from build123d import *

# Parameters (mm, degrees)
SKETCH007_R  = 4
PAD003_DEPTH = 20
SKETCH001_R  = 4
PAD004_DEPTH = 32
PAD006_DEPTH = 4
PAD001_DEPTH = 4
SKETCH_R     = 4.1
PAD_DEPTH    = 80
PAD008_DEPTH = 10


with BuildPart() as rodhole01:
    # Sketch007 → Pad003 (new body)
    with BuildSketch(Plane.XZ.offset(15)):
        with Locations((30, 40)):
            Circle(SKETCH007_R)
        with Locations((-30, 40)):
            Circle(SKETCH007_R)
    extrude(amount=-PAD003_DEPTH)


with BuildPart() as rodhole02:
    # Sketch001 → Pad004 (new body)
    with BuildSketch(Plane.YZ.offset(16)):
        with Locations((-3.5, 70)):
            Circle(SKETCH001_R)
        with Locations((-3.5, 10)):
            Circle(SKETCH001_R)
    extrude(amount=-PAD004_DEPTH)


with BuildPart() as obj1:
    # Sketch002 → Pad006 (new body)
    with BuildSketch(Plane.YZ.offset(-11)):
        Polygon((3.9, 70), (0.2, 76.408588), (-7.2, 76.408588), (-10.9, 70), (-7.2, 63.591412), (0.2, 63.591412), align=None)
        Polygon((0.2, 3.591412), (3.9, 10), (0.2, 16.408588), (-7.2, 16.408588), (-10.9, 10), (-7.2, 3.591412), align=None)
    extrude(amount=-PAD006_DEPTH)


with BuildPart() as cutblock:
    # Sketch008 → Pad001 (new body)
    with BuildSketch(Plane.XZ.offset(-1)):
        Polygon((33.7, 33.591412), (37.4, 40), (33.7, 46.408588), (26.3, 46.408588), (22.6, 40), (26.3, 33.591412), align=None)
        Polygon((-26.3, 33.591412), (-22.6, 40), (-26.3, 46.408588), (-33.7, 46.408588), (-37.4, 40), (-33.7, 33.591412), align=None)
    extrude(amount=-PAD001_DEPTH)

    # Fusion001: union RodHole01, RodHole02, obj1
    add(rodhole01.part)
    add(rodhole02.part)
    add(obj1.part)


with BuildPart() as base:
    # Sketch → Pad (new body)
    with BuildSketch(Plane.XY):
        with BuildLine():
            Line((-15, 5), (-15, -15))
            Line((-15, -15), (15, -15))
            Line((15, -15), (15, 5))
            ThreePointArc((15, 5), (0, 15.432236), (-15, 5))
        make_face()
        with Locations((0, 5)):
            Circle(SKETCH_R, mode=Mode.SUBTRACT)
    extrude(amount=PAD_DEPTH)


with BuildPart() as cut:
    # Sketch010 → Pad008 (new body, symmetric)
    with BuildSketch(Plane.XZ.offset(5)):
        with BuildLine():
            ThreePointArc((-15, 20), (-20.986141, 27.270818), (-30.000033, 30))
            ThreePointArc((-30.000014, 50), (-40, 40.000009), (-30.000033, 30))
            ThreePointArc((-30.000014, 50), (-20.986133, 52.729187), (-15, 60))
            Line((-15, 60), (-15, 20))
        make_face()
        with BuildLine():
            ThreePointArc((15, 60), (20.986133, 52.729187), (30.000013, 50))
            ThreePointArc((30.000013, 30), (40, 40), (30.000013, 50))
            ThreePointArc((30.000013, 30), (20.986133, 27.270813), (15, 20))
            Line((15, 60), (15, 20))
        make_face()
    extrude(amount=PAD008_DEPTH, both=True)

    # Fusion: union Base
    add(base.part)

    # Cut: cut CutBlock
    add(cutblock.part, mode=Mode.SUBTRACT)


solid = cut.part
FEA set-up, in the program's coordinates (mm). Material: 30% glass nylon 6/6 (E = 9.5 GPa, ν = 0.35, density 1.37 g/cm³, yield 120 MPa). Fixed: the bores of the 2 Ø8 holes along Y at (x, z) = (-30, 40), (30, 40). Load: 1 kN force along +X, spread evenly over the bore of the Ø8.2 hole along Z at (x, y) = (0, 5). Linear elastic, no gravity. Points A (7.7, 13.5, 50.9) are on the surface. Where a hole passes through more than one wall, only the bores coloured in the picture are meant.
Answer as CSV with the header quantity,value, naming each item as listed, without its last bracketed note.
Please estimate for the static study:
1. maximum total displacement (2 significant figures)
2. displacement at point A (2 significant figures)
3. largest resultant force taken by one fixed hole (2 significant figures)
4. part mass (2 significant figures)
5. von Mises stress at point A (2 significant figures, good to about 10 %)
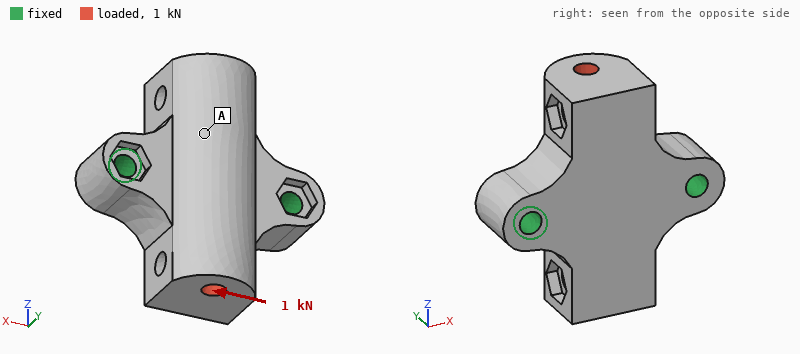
quantity,value
maximum total displacement,10 µm
displacement at point A,5.2 µm
largest resultant force taken by one fixed hole,540 N
part mass,110 g
von Mises stress at point A,0.64 MPa
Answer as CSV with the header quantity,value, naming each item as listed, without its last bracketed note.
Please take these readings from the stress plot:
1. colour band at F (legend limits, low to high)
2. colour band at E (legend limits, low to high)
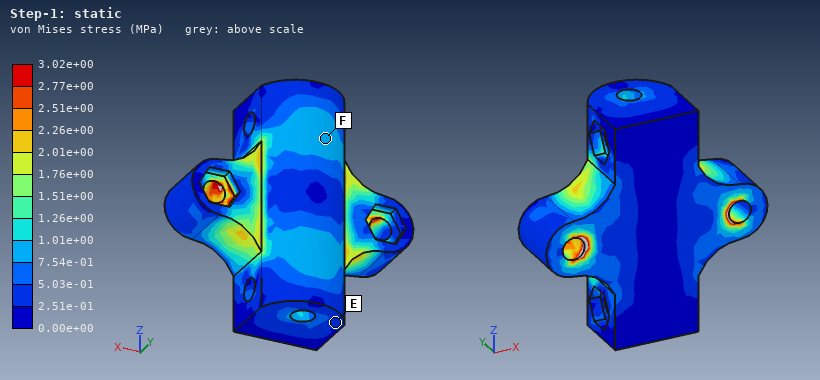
quantity,value
colour band at F,7.54e-01 to 1.01e+00 MPa
colour band at E,2.51e-01 to 5.03e-01 MPa
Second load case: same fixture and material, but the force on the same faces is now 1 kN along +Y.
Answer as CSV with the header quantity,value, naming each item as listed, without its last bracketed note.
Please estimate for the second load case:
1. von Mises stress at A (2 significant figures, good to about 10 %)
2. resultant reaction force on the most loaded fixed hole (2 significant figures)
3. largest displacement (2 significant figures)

quantity,value
von Mises stress at A,2.1 MPa
resultant reaction force on the most loaded fixed hole,540 N
largest displacement,21 µm
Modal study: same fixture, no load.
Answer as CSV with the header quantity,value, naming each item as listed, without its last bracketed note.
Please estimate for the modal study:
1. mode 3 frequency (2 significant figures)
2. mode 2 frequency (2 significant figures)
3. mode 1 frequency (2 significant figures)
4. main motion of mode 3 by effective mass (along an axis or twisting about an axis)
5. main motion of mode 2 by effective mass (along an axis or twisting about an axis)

quantity,value
mode 3 frequency,6700 Hz
mode 2 frequency,4600 Hz
mode 1 frequency,2400 Hz
main motion of mode 3 by effective mass,along Z
main motion of mode 2 by effective mass,along Y
